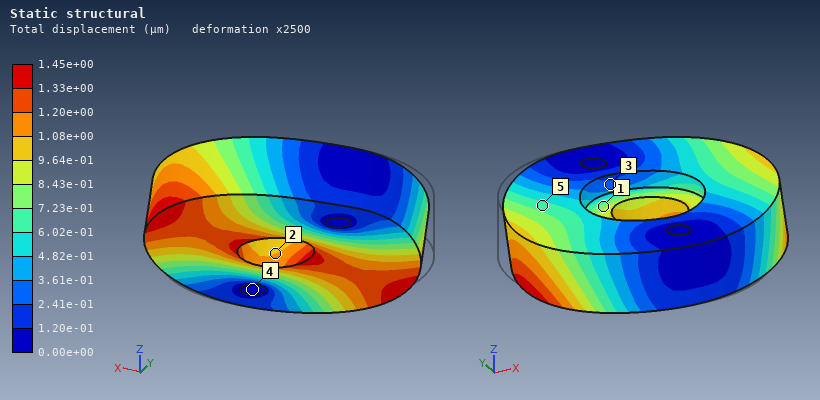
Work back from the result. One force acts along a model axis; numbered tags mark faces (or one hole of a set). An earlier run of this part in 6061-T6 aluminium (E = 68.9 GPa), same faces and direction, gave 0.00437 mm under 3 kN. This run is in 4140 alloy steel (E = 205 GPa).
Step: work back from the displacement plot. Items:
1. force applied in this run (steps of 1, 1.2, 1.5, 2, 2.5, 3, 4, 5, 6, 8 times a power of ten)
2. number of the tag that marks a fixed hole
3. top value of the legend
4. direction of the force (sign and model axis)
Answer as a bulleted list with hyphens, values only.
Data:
- 3 kN
- 4
- 1.45e+00 µm
- +X
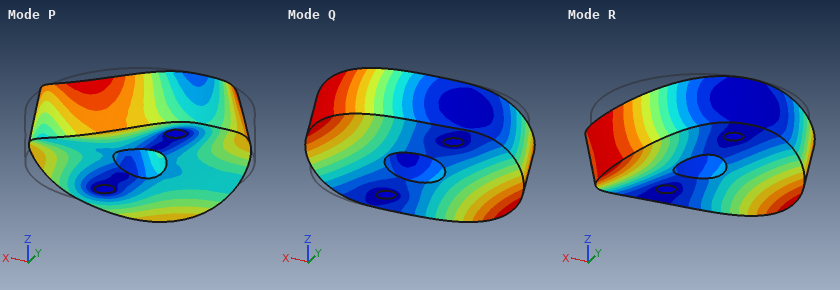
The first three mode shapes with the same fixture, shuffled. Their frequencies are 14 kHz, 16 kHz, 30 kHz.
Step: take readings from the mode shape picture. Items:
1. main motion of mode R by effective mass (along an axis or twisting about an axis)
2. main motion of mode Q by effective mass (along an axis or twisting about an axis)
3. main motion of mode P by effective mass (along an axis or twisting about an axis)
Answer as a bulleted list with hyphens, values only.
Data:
- along Z
- twisting about Y
- twisting about Z
